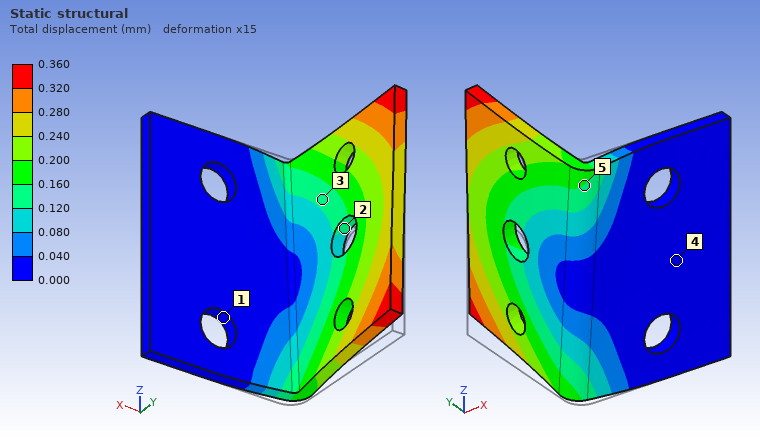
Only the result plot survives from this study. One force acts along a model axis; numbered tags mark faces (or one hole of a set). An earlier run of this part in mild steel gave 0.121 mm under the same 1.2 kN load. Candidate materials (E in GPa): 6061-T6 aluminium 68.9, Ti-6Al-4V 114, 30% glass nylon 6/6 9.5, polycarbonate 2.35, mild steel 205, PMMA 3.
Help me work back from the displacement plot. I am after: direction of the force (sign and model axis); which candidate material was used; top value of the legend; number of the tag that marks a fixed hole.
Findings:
+Z
6061-T6 aluminium
0.360 mm
1
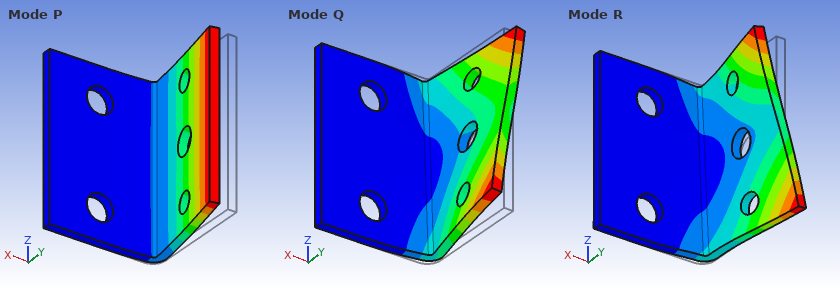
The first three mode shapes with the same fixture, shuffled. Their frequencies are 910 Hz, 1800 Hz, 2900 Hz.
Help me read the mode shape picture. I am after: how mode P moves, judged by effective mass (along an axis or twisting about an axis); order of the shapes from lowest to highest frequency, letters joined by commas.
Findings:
along X
P, Q, R
